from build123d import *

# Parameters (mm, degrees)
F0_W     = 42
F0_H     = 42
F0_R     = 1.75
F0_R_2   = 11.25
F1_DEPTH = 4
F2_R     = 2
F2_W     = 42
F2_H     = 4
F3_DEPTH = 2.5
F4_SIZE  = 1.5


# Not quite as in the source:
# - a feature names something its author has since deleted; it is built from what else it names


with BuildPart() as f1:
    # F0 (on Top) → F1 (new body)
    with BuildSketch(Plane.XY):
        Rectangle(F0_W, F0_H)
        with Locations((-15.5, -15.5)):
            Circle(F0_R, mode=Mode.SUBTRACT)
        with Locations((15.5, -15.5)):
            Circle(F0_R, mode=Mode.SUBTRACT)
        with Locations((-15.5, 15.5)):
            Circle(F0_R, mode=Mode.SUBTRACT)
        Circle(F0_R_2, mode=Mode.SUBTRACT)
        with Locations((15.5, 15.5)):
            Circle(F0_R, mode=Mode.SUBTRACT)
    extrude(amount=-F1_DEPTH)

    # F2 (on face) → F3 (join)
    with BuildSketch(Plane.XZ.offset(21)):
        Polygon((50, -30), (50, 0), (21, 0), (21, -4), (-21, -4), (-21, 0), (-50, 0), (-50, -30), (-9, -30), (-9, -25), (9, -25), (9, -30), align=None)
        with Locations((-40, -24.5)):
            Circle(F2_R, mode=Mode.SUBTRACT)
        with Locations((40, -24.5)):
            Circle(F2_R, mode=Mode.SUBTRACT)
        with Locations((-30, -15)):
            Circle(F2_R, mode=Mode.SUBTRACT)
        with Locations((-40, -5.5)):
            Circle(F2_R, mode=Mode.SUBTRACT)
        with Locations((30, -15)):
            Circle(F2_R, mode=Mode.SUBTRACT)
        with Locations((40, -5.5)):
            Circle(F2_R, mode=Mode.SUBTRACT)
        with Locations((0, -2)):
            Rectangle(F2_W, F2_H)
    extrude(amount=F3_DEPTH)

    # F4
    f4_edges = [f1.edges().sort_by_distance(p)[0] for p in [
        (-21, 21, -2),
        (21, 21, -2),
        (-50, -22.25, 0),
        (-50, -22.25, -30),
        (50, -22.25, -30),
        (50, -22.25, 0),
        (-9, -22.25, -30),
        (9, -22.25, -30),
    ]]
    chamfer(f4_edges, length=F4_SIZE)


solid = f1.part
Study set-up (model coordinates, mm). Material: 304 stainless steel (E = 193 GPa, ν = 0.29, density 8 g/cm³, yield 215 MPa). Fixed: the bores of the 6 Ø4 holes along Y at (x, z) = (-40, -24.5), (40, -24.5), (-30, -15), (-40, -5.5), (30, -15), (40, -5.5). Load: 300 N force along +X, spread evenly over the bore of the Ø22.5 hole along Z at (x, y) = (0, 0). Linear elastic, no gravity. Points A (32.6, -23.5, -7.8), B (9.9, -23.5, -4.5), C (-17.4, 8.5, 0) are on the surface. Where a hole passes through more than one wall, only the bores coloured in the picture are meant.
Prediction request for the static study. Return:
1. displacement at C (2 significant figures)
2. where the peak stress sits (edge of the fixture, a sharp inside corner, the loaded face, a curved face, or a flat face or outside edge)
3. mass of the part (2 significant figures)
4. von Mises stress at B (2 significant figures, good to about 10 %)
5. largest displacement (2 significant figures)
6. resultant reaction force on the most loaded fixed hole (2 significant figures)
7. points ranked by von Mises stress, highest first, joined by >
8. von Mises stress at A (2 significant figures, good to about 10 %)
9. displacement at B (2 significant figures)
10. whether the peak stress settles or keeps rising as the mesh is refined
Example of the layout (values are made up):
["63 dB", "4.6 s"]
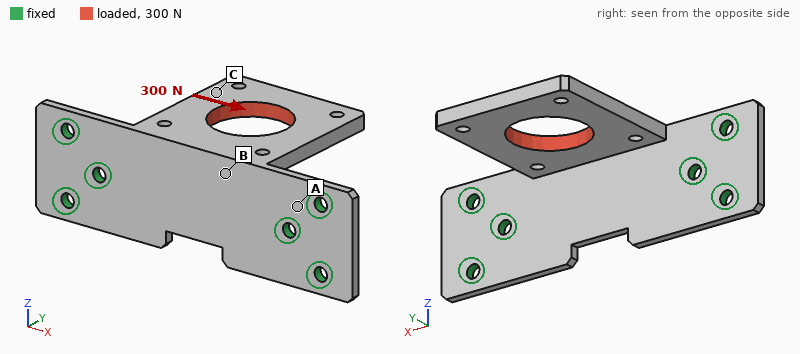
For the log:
["22 µm", "edge of the fixture", "99 g", "9.8 MPa", "31 µm", "140 N", "A > B > C", "28 MPa", "5.1 µm", "keeps rising"]
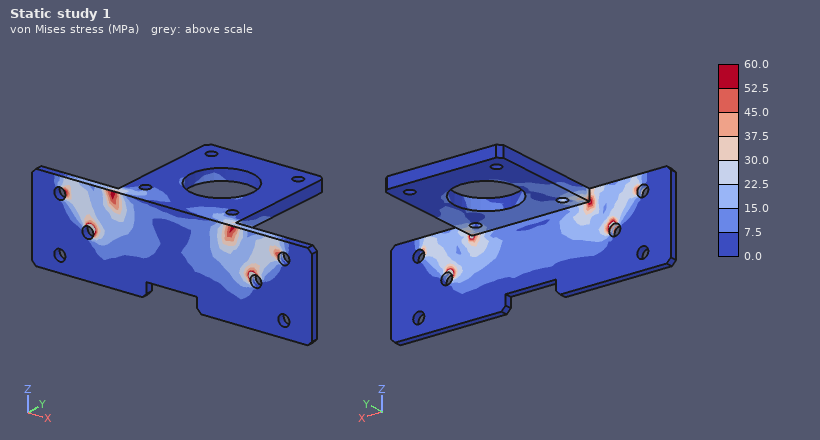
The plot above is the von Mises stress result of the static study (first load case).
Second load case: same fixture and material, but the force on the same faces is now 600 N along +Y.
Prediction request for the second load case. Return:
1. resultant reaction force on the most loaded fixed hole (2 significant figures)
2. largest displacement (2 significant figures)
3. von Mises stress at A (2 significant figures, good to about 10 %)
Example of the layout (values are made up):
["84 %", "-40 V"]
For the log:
["260 N", "0.15 mm", "91 MPa"]
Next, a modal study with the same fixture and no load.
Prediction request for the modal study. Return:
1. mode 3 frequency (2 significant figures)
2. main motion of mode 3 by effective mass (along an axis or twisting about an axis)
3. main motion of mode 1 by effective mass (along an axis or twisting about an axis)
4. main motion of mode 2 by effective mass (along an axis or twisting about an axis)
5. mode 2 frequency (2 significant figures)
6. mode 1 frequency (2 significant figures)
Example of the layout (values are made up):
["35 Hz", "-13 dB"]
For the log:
["3000 Hz", "along Y", "along Z", "along X", "2600 Hz", "830 Hz"]
